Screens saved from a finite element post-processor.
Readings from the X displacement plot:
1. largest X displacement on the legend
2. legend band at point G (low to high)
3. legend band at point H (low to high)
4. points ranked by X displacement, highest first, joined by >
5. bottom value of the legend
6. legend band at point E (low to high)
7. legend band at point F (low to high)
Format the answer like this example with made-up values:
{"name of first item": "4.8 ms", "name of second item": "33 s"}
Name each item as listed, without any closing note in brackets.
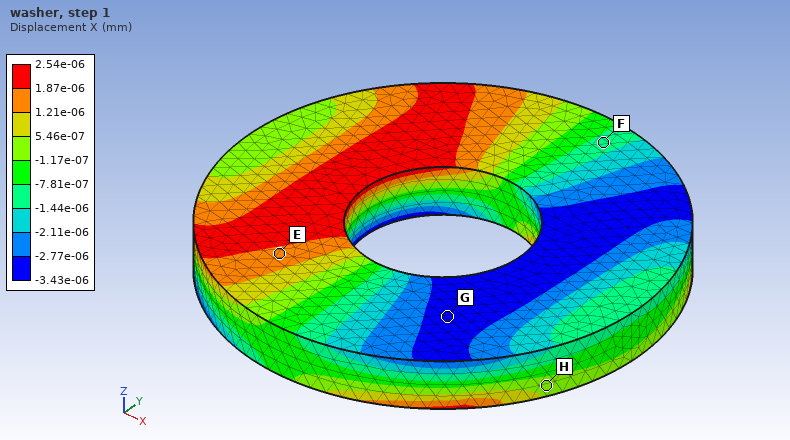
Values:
{"largest X displacement on the legend": "2.54e-06 mm", "legend band at point G": "-3.43e-06 to -2.77e-06 mm", "legend band at point H": "-1.17e-07 to 5.46e-07 mm", "points ranked by X displacement, highest first, joined by >": "E > H > F > G", "bottom value of the legend": "-3.43e-06 mm", "legend band at point E": "1.21e-06 to 1.87e-06 mm", "legend band at point F": "-1.44e-06 to -7.81e-07 mm"}
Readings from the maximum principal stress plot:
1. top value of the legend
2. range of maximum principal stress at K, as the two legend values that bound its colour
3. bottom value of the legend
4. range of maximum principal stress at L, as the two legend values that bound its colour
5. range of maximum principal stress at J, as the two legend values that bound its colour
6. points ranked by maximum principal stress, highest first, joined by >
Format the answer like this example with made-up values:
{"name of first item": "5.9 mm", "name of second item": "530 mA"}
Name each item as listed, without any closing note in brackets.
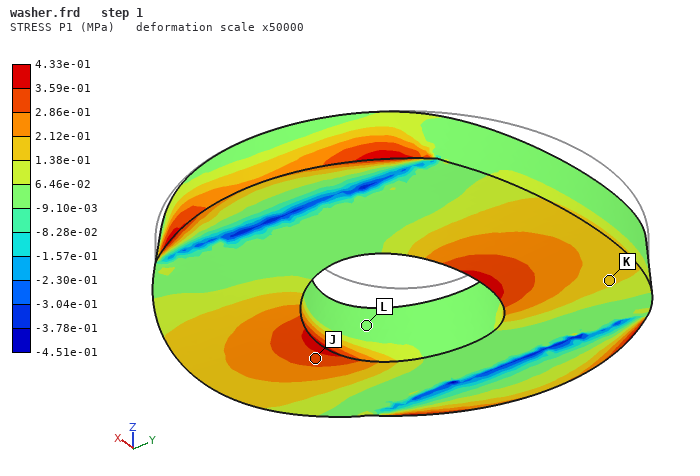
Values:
{"top value of the legend": "4.33e-01 MPa", "range of maximum principal stress at K, as the two legend values that bound its colour": "1.38e-01 to 2.12e-01 MPa", "bottom value of the legend": "-4.51e-01 MPa", "range of maximum principal stress at L, as the two legend values that bound its colour": "-9.10e-03 to 6.46e-02 MPa", "range of maximum principal stress at J, as the two legend values that bound its colour": "2.86e-01 to 3.59e-01 MPa", "points ranked by maximum principal stress, highest first, joined by >": "J > K > L"}
